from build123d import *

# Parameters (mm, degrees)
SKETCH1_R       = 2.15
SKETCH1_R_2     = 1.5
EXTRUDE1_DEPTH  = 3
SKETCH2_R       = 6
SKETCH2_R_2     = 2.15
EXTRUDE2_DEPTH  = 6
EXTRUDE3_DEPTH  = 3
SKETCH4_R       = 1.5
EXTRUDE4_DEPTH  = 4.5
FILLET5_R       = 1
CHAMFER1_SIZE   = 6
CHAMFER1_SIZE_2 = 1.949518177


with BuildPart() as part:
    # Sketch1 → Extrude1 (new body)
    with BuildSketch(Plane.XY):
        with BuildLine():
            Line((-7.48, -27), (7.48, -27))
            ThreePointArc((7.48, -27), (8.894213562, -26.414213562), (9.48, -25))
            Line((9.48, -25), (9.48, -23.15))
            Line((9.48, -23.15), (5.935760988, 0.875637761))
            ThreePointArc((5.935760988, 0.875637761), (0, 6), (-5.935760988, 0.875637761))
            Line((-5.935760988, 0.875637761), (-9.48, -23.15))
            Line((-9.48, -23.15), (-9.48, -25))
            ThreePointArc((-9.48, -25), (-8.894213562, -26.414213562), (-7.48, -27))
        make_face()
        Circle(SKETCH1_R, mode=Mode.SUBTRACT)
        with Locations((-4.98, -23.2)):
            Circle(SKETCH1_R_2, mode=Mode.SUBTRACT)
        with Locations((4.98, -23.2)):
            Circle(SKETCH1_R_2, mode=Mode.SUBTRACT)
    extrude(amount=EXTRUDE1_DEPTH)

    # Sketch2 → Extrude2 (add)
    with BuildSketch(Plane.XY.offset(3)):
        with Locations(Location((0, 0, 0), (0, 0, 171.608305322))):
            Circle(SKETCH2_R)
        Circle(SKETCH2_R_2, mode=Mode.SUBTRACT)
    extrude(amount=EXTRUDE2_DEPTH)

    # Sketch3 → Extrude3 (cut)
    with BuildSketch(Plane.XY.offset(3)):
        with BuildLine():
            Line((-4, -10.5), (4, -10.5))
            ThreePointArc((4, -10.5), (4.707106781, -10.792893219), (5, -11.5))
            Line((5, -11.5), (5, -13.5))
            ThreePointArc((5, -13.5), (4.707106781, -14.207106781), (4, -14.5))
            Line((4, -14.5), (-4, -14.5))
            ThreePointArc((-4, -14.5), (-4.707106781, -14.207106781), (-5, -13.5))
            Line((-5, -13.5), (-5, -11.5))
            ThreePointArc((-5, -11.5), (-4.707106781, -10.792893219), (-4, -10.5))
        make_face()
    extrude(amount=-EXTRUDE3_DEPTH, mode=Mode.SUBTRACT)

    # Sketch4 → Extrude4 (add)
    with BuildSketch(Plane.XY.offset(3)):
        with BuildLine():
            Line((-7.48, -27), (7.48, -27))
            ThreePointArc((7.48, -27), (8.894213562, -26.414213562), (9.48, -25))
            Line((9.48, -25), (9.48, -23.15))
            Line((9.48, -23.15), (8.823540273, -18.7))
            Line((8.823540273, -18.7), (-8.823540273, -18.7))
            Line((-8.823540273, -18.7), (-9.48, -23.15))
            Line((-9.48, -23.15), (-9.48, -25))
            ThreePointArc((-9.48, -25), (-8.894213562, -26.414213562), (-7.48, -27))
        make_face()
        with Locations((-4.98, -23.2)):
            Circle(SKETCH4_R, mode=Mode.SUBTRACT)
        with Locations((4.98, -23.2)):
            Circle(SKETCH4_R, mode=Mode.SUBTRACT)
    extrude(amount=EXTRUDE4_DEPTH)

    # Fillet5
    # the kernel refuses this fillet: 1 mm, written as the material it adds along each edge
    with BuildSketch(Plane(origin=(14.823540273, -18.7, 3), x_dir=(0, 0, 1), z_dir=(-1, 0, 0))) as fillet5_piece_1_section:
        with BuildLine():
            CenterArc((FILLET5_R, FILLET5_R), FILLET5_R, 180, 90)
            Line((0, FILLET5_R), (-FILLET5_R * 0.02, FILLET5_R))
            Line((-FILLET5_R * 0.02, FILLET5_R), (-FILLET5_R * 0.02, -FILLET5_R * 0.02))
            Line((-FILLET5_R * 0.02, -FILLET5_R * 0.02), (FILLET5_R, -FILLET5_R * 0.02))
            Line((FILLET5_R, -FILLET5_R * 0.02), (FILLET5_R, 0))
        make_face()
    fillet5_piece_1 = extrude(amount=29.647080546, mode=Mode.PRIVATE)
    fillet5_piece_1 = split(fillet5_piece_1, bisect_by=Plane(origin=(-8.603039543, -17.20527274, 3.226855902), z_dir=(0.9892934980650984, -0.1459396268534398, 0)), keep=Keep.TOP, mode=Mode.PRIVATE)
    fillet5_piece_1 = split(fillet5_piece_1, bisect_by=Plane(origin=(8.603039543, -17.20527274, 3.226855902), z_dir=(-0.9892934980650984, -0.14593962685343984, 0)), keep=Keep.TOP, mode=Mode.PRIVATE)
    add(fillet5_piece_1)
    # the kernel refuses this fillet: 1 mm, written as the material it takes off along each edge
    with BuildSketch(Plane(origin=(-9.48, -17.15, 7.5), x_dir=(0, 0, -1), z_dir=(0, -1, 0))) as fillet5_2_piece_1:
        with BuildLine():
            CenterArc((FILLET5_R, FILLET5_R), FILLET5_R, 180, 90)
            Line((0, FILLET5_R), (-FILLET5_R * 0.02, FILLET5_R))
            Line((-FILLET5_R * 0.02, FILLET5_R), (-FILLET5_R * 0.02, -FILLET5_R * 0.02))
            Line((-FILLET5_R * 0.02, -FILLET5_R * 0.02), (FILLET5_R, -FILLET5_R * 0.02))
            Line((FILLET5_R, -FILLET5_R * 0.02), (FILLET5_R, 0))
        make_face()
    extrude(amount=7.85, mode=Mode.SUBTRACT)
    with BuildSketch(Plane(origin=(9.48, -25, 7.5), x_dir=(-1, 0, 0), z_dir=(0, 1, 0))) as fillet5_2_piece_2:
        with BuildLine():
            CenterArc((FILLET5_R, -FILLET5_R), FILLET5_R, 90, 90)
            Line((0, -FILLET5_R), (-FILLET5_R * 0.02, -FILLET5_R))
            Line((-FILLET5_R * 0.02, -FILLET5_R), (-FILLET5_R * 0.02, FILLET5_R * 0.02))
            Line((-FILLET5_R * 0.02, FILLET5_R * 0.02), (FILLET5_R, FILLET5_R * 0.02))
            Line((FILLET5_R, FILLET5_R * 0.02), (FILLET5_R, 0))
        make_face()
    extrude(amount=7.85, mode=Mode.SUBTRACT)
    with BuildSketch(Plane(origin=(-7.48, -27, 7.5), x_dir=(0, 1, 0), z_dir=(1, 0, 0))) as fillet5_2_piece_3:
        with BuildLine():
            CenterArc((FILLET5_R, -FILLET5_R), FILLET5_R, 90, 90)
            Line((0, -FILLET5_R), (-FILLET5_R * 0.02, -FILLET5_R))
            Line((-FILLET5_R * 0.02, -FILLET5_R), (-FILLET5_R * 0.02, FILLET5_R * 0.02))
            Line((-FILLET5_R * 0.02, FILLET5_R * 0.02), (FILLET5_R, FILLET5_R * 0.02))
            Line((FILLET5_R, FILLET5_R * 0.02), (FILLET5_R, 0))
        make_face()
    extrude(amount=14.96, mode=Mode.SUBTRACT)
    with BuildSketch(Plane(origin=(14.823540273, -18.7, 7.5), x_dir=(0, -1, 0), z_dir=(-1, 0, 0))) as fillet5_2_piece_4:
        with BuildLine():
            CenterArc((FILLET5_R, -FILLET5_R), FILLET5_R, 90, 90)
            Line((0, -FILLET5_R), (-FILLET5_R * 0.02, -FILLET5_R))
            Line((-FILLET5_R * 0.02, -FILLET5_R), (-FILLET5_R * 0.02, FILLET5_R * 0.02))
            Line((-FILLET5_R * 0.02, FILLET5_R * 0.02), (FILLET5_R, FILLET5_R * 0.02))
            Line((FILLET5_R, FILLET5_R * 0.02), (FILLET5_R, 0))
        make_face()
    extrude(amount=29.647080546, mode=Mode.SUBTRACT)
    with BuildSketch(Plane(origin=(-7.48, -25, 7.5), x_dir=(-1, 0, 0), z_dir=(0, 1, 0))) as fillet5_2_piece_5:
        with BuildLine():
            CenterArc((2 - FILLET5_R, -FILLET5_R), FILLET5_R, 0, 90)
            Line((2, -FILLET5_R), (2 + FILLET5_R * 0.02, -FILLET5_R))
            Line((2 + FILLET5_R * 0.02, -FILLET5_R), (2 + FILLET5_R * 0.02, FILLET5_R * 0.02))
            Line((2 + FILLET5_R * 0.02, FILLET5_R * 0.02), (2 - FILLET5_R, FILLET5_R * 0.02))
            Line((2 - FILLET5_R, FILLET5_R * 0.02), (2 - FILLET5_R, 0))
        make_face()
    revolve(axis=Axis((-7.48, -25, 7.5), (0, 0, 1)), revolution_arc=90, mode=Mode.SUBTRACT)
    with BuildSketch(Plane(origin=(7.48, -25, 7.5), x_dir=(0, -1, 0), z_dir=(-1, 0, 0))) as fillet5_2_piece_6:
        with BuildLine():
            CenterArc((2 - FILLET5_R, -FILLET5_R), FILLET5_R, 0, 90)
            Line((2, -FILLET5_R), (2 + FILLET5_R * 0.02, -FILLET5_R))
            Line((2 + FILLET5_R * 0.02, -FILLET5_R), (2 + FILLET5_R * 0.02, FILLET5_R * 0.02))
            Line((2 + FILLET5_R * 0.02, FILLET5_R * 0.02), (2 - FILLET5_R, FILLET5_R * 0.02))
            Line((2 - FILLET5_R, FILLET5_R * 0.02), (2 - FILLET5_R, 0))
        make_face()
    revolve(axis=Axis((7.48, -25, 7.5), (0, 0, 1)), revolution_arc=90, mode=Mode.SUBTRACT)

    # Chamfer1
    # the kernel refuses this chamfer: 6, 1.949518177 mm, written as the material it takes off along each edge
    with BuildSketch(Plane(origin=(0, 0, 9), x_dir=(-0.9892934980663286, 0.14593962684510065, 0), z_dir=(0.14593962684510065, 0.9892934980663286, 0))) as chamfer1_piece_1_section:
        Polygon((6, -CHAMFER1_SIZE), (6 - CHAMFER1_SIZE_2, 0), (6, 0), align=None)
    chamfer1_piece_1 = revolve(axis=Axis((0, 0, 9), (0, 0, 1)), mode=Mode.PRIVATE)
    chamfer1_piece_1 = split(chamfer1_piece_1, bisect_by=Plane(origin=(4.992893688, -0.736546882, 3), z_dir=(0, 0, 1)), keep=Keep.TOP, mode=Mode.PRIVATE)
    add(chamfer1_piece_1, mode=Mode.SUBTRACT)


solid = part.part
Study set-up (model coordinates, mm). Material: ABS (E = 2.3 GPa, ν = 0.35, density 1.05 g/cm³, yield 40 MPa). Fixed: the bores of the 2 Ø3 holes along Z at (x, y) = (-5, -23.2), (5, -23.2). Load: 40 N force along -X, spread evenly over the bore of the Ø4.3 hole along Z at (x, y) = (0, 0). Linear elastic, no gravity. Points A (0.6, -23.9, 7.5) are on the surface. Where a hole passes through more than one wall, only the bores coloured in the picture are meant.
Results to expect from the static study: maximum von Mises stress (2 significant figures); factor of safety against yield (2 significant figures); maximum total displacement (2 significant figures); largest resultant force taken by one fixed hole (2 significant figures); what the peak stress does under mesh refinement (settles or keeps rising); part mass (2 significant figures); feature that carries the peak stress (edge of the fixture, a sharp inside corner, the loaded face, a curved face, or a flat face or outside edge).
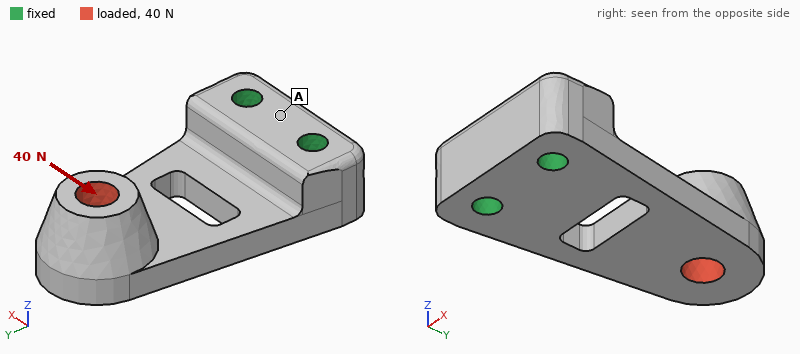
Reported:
25 MPa
1.6
0.26 mm
77 N
settles
2.4 g
a curved face
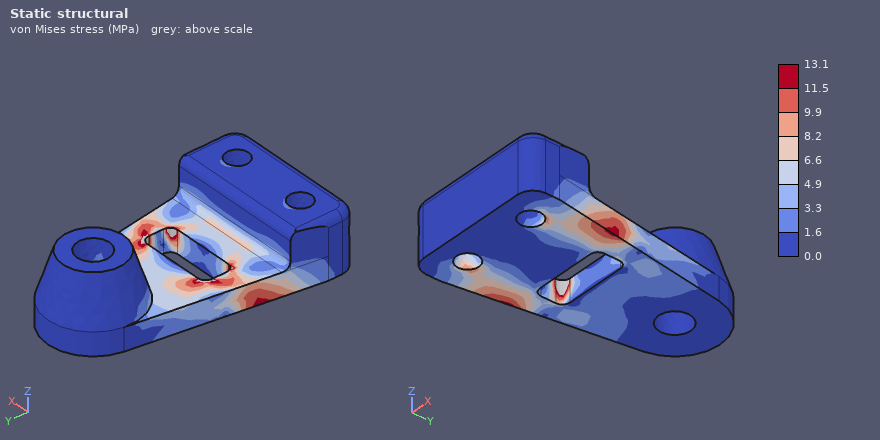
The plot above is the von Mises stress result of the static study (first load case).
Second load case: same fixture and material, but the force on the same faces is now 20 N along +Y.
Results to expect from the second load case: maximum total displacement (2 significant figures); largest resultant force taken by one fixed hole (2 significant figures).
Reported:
0.38 mm
10 N
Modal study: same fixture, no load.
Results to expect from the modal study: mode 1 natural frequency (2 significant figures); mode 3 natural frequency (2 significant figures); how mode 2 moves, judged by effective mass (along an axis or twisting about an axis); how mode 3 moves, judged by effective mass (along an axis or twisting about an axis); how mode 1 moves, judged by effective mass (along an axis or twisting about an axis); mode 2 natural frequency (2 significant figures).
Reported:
720 Hz
4100 Hz
along X
along X
along Z
2600 Hz
